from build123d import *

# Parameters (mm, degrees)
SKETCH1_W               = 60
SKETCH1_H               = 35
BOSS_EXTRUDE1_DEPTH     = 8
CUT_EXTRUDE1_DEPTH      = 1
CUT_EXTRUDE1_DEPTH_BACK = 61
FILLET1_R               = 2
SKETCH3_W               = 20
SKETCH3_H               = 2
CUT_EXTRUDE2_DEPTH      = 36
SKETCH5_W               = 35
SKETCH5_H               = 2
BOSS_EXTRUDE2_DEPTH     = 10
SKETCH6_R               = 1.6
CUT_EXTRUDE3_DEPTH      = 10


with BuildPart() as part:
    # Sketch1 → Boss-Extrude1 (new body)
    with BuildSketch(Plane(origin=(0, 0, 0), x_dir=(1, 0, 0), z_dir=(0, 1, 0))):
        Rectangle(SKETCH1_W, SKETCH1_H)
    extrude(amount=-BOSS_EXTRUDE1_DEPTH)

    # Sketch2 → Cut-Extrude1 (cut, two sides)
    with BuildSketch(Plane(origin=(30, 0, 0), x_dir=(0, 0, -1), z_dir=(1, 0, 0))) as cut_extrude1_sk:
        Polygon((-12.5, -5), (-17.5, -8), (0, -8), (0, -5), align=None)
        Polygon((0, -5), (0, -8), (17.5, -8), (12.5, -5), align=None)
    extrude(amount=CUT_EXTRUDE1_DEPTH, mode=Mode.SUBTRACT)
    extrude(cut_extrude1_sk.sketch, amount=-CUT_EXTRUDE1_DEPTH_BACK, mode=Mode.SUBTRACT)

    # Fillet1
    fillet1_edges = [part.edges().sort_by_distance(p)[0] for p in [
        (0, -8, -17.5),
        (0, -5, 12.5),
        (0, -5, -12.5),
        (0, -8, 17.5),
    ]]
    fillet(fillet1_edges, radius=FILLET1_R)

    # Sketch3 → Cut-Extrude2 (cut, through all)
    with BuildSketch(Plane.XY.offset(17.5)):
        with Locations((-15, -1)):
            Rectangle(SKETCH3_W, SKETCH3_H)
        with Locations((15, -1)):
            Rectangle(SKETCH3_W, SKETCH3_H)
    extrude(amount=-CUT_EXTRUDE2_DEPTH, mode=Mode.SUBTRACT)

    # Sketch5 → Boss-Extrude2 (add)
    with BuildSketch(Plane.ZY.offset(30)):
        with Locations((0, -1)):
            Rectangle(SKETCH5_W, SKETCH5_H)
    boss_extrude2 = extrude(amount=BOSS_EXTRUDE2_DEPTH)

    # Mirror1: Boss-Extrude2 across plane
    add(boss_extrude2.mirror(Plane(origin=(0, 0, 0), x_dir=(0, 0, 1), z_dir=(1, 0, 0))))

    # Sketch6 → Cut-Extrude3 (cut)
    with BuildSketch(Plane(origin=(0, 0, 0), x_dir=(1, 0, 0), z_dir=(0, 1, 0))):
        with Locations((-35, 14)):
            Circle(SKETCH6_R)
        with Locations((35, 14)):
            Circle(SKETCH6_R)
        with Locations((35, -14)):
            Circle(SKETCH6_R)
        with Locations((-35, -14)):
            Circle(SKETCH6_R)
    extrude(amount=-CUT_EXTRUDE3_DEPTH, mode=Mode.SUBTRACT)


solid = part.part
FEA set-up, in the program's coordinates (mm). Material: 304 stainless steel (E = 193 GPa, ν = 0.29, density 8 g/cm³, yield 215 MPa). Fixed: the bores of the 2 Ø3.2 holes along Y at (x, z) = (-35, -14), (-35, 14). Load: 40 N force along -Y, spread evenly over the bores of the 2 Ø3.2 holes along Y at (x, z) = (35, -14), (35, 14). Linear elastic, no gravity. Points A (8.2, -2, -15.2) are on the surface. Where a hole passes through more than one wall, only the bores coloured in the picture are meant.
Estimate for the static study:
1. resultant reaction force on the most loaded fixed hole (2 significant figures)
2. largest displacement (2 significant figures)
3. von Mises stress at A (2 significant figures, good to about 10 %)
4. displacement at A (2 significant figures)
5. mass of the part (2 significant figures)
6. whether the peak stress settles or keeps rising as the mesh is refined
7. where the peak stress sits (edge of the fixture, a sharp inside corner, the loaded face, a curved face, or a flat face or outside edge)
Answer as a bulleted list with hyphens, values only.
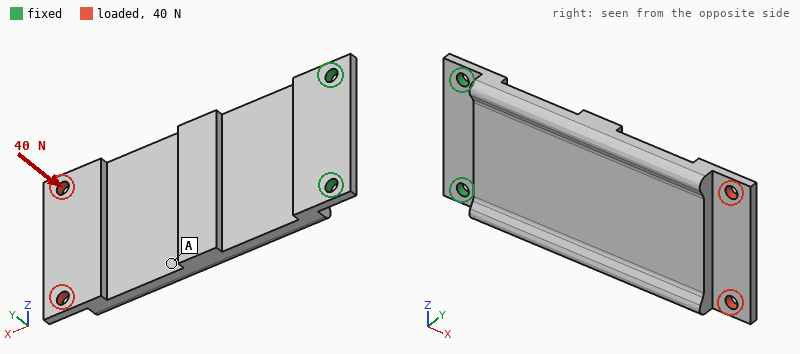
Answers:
- 53 N
- 0.43 mm
- 15 MPa
- 0.21 mm
- 77 g
- keeps rising
- edge of the fixture
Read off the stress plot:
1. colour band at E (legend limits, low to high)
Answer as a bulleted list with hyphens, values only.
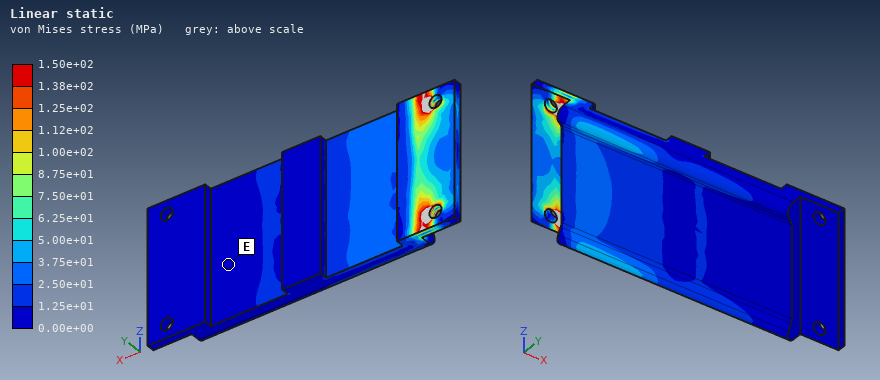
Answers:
- 0.00e+00 to 1.25e+01 MPa
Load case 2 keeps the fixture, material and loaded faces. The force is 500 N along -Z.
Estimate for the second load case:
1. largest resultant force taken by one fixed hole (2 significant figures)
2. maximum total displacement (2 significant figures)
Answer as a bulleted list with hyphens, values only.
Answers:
- 1.2 kN
- 93 µm
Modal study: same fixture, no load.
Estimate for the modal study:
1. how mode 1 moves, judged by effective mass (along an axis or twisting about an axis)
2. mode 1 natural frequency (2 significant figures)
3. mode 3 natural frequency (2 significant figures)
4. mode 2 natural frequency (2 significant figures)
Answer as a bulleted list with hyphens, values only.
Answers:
- along Y
- 340 Hz
- 2700 Hz
- 2000 Hz
